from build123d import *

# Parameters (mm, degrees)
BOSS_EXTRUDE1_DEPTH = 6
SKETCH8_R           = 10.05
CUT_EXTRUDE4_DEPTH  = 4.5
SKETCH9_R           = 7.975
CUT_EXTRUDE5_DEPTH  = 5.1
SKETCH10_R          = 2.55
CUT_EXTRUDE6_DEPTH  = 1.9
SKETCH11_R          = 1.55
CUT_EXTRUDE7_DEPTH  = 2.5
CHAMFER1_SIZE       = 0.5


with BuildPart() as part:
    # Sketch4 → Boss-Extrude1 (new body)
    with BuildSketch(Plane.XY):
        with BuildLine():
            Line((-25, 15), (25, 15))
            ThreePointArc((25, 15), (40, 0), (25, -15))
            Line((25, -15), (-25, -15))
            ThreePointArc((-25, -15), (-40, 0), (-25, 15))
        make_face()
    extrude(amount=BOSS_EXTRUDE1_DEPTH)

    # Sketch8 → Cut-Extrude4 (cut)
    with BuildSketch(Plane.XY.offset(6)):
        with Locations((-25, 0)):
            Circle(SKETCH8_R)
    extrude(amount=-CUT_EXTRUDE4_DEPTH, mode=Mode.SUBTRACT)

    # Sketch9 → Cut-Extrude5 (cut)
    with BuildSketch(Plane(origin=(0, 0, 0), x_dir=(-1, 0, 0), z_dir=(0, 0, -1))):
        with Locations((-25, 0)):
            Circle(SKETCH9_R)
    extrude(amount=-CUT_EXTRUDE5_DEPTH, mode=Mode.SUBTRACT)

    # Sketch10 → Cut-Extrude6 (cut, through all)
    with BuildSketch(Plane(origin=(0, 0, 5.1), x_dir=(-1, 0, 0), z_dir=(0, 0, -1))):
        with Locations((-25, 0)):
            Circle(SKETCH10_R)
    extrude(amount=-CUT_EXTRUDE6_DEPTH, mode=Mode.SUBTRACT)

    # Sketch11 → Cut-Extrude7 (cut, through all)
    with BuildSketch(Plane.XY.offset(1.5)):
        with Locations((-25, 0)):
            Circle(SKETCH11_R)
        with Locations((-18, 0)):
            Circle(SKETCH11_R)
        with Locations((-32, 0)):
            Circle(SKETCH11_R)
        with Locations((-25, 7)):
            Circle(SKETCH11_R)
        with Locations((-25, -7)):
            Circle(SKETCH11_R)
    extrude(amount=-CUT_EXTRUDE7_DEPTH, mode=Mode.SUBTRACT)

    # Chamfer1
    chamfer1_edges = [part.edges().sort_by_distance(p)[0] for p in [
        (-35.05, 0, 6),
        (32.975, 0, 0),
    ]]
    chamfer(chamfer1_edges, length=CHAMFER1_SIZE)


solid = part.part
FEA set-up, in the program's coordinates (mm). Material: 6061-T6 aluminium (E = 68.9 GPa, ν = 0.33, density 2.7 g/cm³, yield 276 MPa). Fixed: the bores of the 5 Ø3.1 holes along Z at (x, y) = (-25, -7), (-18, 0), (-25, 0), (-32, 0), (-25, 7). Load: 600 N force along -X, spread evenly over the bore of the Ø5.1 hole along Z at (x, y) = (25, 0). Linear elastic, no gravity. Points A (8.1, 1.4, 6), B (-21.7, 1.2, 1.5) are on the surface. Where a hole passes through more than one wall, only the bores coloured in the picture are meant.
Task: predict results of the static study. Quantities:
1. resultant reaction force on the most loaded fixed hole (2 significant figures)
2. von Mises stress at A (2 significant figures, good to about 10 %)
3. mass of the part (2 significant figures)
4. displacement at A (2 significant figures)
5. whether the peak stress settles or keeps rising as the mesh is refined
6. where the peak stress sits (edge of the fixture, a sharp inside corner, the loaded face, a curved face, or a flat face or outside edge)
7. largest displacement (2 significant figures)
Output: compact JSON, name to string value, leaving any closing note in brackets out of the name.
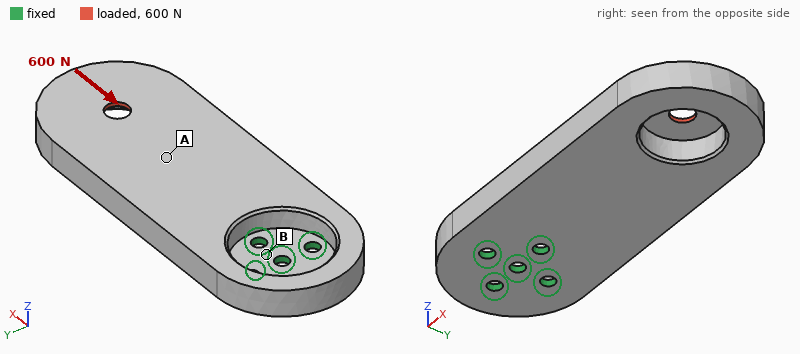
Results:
{"resultant reaction force on the most loaded fixed hole": "260 N", "von Mises stress at A": "11 MPa", "mass of the part": "29 g", "displacement at A": "0.056 mm", "whether the peak stress settles or keeps rising as the mesh is refined": "keeps rising", "where the peak stress sits": "edge of the fixture", "largest displacement": "0.15 mm"}
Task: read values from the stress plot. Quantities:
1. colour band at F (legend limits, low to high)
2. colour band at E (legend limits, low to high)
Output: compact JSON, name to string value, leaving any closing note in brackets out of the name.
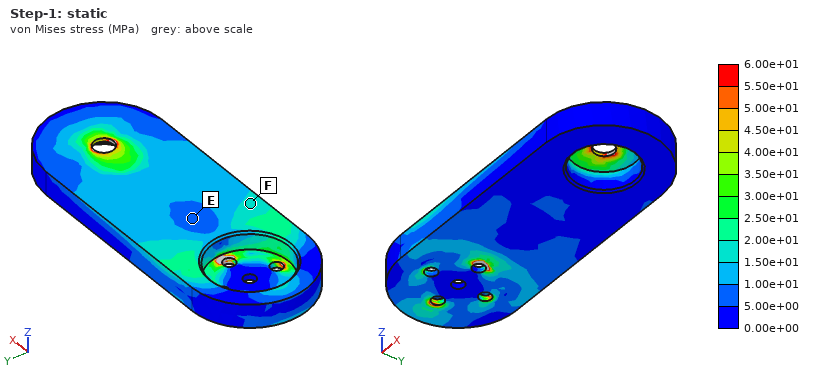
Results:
{"colour band at F": "1.50e+01 to 2.00e+01 MPa", "colour band at E": "5.00e+00 to 1.00e+01 MPa"}
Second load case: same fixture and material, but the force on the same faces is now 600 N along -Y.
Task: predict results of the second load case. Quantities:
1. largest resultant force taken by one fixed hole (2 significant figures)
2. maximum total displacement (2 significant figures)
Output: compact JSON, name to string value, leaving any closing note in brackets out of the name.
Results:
{"largest resultant force taken by one fixed hole": "1.1 kN", "maximum total displacement": "96 µm"}
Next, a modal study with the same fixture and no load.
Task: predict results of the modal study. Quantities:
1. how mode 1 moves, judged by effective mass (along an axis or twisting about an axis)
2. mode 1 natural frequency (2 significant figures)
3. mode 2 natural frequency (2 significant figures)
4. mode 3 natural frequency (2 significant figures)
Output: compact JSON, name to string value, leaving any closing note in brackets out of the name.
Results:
{"how mode 1 moves, judged by effective mass": "along Z", "mode 1 natural frequency": "1100 Hz", "mode 2 natural frequency": "4100 Hz", "mode 3 natural frequency": "4200 Hz"}
